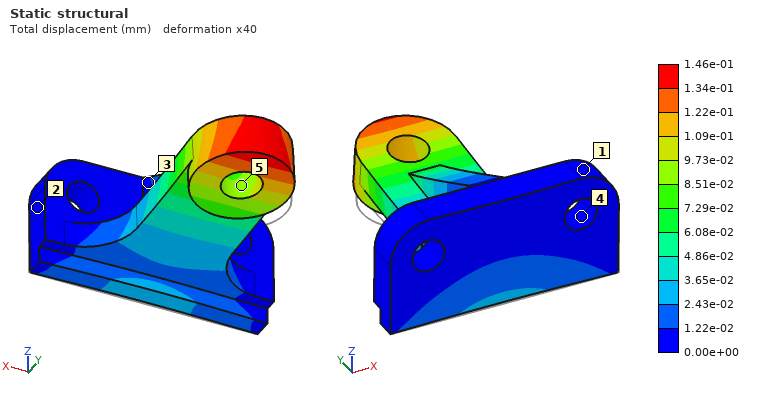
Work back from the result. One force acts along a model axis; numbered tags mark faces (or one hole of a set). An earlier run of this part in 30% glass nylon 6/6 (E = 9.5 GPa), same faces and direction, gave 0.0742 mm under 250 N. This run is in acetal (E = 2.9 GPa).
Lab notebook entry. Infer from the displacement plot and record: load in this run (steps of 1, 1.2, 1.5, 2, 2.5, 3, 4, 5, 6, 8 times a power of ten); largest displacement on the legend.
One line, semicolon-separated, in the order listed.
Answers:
150 N; 1.46e-01 mm
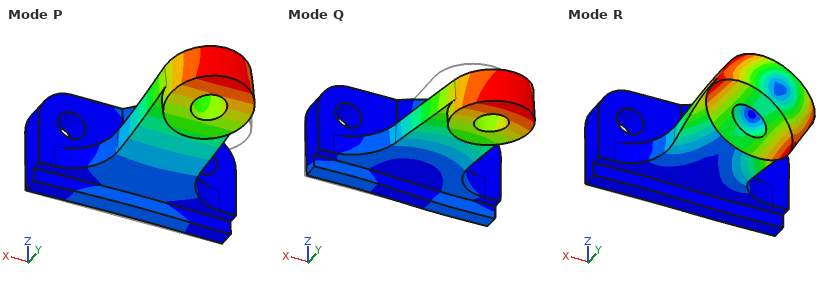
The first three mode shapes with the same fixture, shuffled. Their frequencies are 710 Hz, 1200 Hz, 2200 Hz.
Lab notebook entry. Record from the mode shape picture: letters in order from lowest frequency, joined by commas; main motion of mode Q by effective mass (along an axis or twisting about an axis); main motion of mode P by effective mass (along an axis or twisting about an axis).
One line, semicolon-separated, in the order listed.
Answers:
P, Q, R; along X; along Z
